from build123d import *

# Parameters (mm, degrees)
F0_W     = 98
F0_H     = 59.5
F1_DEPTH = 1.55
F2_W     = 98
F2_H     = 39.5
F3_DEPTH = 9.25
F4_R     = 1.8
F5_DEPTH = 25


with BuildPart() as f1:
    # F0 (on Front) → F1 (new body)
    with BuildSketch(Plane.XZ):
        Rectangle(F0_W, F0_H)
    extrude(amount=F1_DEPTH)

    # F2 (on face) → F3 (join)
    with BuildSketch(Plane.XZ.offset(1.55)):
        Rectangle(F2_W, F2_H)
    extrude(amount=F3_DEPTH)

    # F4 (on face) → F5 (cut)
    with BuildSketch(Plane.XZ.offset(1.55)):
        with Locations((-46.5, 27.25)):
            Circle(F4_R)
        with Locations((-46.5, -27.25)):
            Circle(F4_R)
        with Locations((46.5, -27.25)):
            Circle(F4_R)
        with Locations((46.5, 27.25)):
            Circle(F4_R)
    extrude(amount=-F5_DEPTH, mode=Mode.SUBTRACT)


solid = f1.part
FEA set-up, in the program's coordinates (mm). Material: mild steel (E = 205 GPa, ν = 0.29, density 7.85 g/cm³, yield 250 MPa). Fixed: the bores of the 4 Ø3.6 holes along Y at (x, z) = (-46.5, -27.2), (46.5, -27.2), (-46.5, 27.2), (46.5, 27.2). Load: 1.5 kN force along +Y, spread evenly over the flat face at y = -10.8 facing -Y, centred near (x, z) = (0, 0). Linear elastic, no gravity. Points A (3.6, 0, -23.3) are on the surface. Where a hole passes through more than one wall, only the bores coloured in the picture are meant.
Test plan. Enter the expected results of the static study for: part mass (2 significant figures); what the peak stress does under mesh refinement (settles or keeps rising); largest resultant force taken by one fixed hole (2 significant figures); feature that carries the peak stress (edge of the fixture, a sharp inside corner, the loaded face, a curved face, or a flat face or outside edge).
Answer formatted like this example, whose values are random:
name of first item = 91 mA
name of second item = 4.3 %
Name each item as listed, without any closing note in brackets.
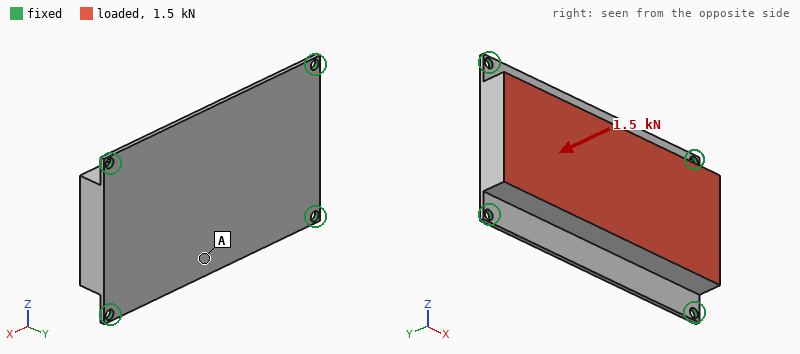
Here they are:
part mass = 350 g
what the peak stress does under mesh refinement = keeps rising
largest resultant force taken by one fixed hole = 570 N
feature that carries the peak stress = edge of the fixture
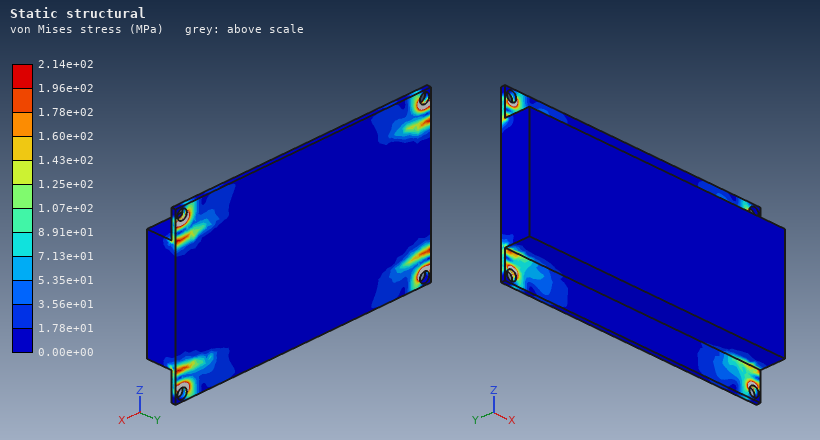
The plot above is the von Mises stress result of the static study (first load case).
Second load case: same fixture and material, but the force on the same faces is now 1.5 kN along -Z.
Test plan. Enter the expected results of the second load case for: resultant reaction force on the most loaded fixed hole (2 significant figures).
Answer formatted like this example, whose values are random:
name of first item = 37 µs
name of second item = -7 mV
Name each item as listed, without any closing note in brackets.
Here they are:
resultant reaction force on the most loaded fixed hole = 440 N
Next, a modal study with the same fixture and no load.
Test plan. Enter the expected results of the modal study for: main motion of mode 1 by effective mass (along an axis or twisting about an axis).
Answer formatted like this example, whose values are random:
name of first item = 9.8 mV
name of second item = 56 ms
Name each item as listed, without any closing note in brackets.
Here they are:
main motion of mode 1 by effective mass = along Y
